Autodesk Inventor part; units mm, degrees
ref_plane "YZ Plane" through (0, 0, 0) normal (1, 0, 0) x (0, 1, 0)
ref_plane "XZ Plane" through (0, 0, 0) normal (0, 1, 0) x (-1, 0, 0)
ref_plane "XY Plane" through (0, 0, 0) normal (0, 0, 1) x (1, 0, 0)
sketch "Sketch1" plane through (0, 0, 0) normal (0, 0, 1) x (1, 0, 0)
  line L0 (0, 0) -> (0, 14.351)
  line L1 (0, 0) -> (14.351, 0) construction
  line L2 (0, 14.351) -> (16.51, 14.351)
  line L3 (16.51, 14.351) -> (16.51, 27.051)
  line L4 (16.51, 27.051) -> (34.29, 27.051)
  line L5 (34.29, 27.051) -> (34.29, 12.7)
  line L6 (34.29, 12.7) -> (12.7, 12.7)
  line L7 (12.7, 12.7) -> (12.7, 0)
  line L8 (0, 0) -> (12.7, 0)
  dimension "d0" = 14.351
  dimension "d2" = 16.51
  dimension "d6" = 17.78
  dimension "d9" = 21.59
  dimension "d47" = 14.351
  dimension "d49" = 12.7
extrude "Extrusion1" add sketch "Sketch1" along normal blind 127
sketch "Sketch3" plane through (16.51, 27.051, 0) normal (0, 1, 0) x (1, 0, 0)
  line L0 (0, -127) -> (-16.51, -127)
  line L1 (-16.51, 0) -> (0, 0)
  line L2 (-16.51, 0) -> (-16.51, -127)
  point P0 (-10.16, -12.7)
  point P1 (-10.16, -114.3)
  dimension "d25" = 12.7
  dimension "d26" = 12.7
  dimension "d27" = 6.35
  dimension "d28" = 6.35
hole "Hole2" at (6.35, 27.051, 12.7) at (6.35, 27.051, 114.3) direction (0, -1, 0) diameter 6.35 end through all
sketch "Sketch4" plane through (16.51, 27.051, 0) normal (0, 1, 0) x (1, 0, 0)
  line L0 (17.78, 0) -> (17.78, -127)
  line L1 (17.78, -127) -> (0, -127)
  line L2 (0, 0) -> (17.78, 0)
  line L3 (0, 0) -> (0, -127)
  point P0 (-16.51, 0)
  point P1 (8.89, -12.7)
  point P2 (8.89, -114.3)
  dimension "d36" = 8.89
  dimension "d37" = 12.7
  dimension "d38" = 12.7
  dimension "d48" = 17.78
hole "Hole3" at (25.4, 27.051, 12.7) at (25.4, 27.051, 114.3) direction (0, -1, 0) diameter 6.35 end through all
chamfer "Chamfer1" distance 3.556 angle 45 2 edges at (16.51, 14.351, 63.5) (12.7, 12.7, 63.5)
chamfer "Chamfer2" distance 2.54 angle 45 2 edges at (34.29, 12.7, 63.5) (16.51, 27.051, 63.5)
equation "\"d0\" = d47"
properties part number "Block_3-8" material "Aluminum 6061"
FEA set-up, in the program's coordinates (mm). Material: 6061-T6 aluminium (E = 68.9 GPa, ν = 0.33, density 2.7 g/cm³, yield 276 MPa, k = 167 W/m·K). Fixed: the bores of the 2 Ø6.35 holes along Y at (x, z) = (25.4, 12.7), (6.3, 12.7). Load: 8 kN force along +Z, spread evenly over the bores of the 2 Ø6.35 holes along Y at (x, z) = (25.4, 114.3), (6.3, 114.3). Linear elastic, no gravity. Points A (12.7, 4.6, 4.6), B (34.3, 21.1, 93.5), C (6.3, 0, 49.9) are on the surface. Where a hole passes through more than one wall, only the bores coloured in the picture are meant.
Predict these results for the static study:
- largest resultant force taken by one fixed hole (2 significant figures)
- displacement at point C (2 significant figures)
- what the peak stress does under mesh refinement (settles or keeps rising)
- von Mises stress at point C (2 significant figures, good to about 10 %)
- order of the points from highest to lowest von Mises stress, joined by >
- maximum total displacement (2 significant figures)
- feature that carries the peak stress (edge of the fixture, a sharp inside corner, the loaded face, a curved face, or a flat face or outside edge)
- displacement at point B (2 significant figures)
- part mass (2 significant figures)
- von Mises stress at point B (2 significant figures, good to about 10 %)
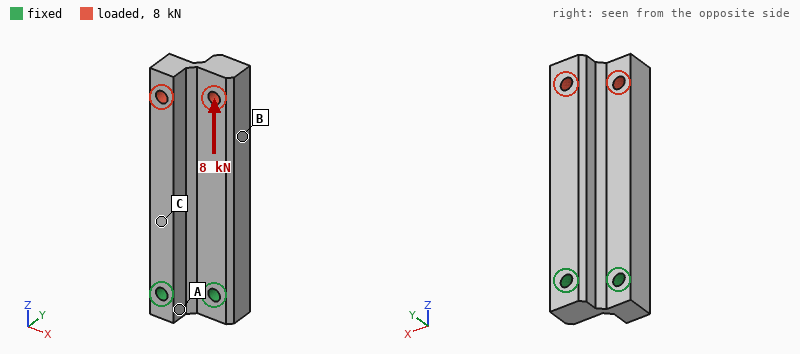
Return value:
4.0 kN
12 µm
keeps rising
21 MPa
C > B > A
38 µm
edge of the fixture
18 µm
150 g
14 MPa
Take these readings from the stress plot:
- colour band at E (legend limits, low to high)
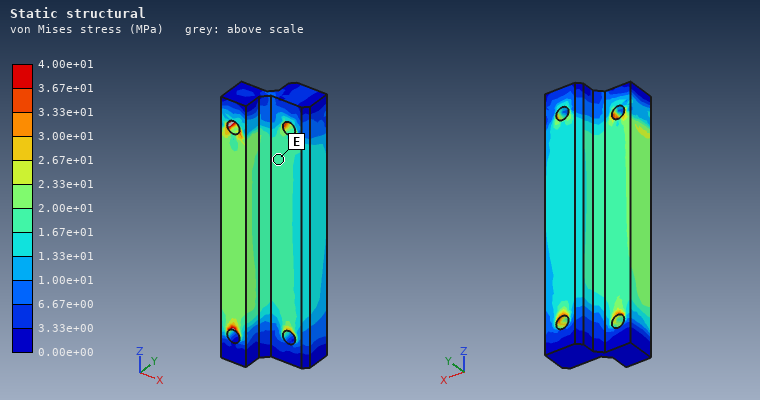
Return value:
1.67e+01 to 2.00e+01 MPa
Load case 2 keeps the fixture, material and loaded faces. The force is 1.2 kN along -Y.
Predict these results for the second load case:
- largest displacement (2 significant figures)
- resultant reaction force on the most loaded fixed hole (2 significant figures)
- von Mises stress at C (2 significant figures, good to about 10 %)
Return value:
0.83 mm
2.0 kN
65 MPa
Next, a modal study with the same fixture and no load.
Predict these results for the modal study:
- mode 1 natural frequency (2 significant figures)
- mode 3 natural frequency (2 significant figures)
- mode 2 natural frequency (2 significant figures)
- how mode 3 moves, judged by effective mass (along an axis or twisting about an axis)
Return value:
890 Hz
3400 Hz
2300 Hz
twisting about Z
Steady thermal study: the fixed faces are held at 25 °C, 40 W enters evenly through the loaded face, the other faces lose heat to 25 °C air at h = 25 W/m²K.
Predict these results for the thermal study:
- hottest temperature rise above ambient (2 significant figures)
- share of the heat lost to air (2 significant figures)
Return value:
48 K
21 %
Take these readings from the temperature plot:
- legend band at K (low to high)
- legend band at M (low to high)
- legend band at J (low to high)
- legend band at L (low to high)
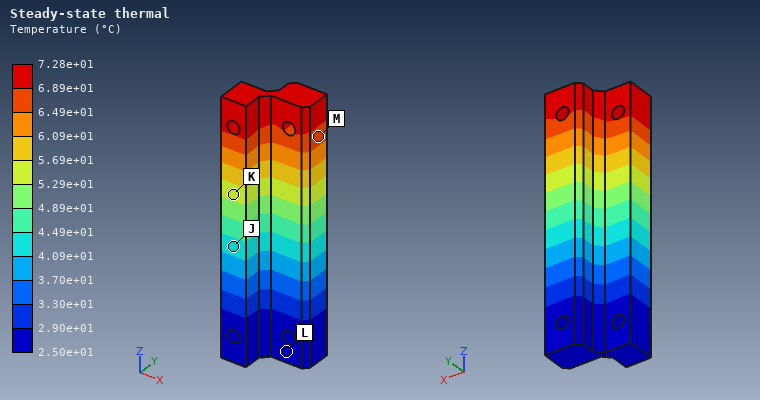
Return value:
5.29e+01 to 5.69e+01 °C
6.49e+01 to 6.89e+01 °C
4.09e+01 to 4.49e+01 °C
2.50e+01 to 2.90e+01 °C
